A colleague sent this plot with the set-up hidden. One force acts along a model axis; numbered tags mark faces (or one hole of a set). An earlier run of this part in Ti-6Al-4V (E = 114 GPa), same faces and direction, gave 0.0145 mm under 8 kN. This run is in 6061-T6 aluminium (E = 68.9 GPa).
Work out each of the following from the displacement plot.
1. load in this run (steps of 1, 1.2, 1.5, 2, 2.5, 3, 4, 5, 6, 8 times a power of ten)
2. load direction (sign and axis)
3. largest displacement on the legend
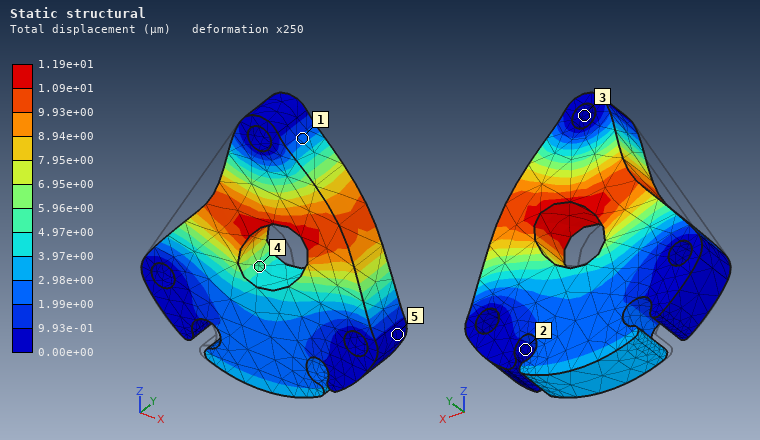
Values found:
4 kN
+X
1.19e+01 µm
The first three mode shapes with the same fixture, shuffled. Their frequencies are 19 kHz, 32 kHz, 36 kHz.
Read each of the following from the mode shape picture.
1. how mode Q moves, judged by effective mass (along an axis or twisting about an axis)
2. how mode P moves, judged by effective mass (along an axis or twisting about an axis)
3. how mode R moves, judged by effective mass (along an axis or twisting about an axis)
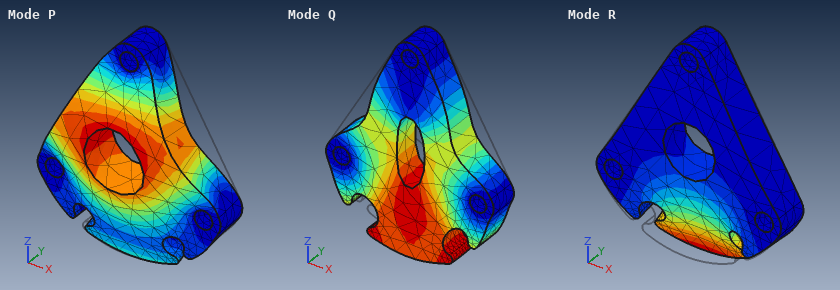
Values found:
along Z
along Y
along Y
